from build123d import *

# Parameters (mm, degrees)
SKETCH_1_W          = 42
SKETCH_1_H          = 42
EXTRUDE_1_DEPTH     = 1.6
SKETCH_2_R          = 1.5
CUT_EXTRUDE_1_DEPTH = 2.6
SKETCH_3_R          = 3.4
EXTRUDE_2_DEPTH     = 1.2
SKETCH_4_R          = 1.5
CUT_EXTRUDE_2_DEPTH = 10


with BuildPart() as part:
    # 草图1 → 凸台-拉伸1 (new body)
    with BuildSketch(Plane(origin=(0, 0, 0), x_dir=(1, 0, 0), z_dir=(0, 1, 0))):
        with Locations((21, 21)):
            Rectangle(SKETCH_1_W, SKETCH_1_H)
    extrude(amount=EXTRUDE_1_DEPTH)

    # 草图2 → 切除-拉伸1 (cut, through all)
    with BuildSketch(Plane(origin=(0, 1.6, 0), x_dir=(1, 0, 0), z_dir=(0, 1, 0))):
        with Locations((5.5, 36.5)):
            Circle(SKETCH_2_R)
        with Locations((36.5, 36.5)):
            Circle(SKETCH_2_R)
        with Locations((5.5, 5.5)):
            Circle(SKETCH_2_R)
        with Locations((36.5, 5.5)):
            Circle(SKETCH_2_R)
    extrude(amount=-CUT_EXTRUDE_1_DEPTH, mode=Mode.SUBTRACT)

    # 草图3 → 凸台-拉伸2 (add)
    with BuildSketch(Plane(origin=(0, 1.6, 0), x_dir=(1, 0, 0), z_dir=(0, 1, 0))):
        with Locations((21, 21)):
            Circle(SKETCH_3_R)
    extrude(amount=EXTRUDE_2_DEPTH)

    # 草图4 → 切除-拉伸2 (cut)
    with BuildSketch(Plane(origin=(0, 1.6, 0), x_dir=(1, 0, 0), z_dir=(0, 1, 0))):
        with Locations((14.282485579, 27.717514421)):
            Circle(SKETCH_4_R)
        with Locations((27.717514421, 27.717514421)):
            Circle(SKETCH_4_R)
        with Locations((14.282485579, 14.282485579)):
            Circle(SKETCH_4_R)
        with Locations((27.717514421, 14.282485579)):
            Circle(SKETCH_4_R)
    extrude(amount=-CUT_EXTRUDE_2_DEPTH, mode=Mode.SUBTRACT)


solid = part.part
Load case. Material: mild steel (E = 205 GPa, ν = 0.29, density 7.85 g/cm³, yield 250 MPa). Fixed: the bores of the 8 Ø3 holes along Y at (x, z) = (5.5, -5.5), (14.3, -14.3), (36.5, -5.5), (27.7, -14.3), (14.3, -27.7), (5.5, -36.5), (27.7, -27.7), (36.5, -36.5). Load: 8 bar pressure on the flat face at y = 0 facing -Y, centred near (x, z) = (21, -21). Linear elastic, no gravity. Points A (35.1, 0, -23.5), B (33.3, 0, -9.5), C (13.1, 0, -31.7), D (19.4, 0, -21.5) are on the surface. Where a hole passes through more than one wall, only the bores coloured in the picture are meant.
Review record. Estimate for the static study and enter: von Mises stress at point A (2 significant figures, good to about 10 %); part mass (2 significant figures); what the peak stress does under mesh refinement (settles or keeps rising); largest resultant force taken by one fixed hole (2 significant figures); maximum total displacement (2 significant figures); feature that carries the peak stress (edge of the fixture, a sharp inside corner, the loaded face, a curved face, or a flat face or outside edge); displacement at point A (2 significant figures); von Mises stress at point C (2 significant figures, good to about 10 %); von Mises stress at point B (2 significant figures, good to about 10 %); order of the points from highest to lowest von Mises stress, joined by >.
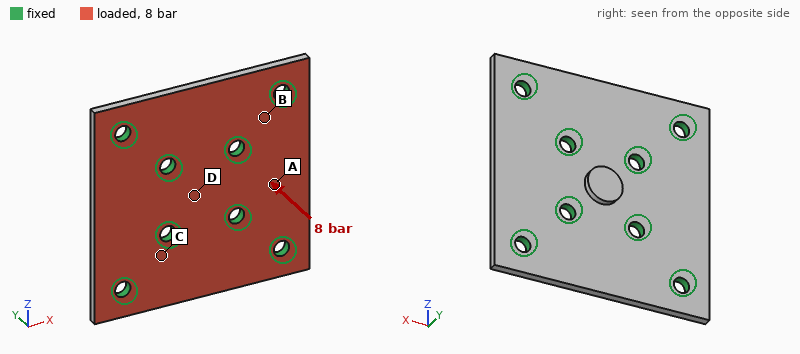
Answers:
22 MPa
22 g
keeps rising
170 N
17 µm
edge of the fixture
6.9 µm
40 MPa
48 MPa
B > C > A > D
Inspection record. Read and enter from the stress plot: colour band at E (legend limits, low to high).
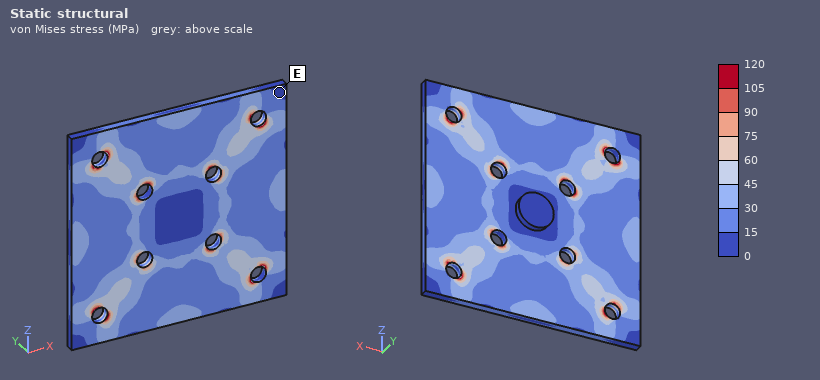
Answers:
0 to 15 MPa
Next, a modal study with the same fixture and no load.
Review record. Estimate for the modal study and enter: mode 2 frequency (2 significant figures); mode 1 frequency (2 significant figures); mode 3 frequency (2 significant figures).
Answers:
13 kHz
13 kHz
13 kHz
